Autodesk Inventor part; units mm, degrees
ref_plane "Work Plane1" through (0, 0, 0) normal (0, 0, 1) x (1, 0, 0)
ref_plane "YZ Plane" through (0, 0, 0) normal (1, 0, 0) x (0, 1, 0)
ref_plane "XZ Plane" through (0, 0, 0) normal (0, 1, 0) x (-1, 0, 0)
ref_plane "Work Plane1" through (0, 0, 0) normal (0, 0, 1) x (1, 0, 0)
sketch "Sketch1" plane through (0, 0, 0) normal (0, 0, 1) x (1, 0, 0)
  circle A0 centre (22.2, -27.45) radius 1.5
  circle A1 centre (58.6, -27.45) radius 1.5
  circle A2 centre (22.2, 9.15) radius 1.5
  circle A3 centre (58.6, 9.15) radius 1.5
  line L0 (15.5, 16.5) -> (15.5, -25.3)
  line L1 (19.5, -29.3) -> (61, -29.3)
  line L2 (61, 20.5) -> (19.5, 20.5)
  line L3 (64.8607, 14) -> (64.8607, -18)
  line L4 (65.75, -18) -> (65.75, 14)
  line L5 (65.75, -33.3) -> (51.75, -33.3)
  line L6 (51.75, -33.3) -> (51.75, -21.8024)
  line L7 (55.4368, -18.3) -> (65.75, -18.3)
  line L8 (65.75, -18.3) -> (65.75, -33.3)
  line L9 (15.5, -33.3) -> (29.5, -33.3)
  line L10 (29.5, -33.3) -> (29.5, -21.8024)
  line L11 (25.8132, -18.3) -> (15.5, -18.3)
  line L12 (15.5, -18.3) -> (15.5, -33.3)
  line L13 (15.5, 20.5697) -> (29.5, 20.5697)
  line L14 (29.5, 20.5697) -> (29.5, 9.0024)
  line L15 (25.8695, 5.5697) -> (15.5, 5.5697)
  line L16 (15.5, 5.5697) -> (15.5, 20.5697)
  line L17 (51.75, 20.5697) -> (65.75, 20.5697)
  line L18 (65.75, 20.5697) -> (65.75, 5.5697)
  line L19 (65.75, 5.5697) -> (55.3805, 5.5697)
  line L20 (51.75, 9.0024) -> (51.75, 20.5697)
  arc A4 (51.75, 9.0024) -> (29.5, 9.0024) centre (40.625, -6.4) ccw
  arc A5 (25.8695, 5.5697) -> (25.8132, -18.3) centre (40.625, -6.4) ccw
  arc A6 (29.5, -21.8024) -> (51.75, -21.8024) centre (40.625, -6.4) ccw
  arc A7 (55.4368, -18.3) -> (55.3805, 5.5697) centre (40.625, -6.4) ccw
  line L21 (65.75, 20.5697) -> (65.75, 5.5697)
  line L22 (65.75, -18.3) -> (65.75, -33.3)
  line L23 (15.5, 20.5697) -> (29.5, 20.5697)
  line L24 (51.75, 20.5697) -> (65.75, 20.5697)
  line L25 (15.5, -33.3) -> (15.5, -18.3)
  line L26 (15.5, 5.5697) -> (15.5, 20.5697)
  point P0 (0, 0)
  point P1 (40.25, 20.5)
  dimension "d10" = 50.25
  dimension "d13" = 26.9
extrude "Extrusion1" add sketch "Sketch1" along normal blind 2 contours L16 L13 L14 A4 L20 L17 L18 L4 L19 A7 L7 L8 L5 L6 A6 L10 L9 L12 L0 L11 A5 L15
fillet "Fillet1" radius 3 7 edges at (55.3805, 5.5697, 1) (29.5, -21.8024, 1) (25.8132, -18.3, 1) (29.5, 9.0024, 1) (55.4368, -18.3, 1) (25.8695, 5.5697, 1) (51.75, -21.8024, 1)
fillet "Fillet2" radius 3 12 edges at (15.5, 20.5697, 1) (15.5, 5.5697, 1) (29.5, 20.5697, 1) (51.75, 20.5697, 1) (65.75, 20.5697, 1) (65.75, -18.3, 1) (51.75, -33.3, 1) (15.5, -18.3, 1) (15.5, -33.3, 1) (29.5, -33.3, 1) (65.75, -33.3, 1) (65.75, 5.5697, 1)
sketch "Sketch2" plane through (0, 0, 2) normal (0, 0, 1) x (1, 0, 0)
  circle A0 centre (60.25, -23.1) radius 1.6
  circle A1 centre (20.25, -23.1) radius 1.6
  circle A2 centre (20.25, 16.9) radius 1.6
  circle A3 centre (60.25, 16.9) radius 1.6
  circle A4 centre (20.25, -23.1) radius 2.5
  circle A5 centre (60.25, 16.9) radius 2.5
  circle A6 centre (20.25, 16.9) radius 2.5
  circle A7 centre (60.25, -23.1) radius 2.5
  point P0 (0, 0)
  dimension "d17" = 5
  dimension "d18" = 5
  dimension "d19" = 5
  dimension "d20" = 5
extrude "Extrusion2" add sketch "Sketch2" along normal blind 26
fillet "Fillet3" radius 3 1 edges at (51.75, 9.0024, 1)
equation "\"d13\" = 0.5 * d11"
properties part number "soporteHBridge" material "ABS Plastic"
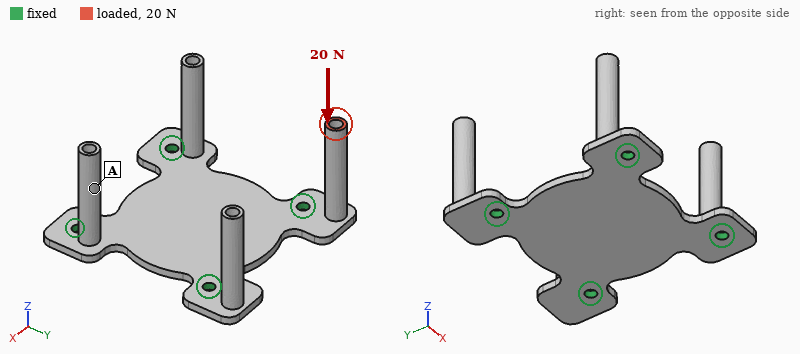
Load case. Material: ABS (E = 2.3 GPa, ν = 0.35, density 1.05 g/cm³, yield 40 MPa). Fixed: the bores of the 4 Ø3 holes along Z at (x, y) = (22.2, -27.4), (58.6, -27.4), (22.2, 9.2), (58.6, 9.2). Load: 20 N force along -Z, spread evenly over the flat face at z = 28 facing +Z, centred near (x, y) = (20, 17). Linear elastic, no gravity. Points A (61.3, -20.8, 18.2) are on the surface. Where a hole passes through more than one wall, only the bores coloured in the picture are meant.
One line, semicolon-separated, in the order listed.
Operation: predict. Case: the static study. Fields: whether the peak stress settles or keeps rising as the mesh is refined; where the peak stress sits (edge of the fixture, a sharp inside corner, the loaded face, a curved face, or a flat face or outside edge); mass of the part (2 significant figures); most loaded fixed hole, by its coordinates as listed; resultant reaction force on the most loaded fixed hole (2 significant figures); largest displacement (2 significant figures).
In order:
keeps rising; edge of the fixture; 5.3 g; (22.2, 9.2); 21 N; 0.78 mm
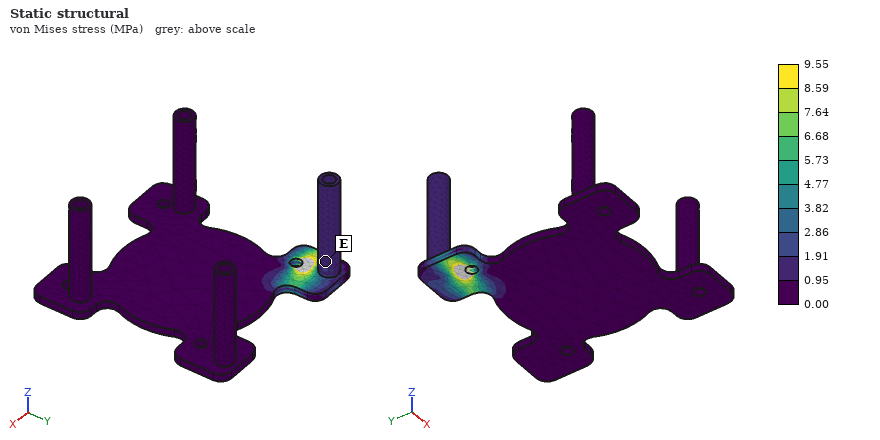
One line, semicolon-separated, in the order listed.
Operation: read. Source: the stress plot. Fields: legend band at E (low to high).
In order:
0.95 to 1.91 MPa
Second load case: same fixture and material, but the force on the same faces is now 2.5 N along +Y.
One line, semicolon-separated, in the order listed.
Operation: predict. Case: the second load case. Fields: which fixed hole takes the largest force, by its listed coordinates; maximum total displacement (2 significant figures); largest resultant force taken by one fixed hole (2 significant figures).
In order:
(22.2, 9.2); 0.88 mm; 2.7 N
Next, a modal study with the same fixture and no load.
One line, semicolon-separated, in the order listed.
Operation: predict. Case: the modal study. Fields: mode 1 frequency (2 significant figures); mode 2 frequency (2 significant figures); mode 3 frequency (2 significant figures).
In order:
820 Hz; 830 Hz; 990 Hz
